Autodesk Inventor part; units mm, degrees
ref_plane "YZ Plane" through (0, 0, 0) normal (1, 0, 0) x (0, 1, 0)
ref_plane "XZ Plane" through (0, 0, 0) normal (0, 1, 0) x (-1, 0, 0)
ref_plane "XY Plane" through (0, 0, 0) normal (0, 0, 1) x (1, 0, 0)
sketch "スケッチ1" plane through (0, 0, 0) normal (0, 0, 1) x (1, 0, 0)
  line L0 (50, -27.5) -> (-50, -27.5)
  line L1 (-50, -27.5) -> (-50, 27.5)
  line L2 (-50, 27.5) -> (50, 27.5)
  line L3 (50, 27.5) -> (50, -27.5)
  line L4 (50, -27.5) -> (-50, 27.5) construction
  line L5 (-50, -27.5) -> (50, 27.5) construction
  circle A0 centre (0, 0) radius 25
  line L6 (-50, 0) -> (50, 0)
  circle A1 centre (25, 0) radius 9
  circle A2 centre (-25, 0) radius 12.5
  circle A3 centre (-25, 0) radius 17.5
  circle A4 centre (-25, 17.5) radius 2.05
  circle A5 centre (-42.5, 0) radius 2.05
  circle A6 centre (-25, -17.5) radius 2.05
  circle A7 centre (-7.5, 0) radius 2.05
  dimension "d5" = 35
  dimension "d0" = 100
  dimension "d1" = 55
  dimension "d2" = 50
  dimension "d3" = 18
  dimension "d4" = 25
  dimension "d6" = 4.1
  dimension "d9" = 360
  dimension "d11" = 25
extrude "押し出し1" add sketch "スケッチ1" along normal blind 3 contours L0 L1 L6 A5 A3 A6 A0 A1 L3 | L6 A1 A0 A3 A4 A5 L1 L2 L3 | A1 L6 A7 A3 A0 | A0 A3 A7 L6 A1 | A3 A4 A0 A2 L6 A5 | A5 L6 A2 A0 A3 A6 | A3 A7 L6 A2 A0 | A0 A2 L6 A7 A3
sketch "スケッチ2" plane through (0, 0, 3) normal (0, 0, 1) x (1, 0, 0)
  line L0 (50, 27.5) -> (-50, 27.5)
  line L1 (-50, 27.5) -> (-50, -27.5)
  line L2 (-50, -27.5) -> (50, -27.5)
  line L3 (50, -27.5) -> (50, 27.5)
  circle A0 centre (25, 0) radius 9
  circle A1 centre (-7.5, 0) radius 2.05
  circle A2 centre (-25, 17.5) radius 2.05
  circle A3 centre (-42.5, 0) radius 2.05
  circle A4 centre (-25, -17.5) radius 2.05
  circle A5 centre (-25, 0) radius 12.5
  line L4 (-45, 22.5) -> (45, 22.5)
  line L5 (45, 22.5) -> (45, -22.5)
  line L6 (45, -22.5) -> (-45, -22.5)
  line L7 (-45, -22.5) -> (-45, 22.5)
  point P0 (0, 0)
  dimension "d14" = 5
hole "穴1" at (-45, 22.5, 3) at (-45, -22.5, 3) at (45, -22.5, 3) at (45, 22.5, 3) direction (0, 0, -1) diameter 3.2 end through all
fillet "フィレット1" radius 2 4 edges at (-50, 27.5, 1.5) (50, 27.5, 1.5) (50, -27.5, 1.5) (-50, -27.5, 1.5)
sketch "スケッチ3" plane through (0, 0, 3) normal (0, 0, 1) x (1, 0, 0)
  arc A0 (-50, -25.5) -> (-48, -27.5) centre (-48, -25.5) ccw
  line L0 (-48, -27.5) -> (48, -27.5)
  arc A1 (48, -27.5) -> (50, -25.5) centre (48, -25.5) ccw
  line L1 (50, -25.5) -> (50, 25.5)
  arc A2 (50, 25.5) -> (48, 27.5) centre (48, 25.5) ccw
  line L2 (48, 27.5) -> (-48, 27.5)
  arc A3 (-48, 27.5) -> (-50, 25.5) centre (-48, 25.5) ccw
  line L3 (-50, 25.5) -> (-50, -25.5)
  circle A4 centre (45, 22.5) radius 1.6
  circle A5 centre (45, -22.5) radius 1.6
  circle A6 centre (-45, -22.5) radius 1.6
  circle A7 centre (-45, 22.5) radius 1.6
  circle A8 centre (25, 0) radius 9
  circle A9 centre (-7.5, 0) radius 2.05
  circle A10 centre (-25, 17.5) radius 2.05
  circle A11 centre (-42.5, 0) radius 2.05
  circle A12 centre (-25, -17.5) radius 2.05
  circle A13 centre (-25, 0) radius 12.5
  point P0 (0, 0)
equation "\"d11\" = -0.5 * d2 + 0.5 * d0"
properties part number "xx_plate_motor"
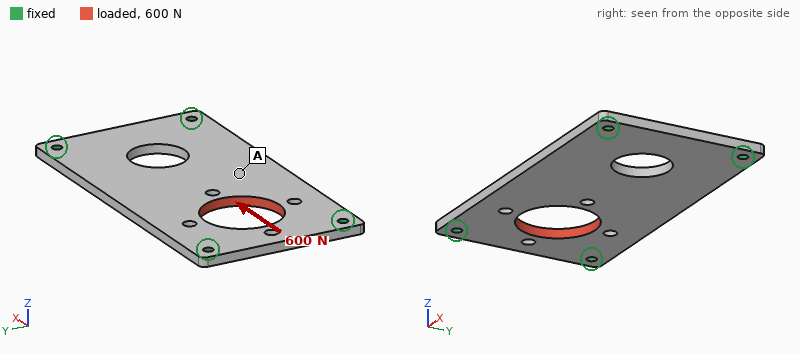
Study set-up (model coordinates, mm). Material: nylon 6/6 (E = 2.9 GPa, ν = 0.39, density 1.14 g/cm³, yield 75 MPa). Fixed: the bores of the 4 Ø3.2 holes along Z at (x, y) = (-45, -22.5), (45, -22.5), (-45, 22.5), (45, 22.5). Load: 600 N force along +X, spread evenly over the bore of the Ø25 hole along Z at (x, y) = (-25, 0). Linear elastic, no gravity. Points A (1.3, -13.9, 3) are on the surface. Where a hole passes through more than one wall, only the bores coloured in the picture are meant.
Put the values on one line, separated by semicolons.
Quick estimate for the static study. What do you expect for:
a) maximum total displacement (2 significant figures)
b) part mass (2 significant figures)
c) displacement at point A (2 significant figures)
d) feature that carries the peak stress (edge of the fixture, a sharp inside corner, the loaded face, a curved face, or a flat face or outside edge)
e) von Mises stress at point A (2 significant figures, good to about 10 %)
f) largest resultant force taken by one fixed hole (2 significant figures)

87 µm; 16 g; 30 µm; edge of the fixture; 1.8 MPa; 210 N
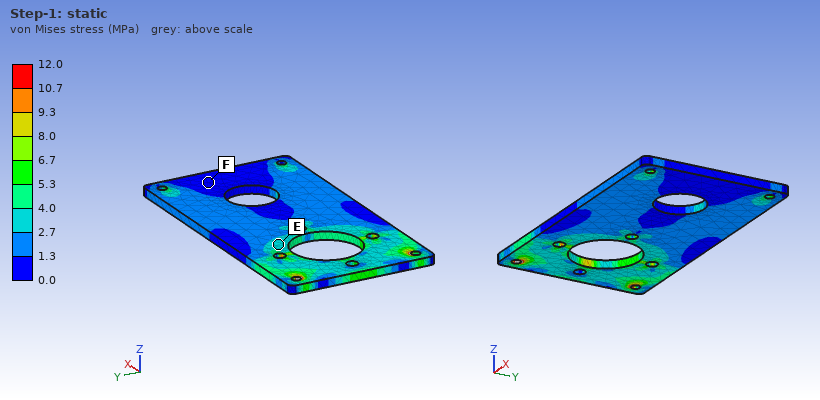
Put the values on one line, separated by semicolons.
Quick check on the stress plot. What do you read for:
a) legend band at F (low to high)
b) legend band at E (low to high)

0.0 to 1.3 MPa; 2.7 to 4.0 MPa
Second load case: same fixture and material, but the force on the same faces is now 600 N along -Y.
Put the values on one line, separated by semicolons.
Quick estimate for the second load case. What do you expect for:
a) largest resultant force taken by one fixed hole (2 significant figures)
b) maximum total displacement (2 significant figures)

230 N; 0.15 mm
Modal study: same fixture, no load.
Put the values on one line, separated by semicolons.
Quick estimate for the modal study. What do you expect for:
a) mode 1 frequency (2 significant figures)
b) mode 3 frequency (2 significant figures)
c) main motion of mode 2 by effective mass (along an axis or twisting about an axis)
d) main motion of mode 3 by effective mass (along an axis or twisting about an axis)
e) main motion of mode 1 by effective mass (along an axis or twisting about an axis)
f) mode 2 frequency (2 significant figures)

540 Hz; 1500 Hz; twisting about X; twisting about Y; along Z; 820 Hz
